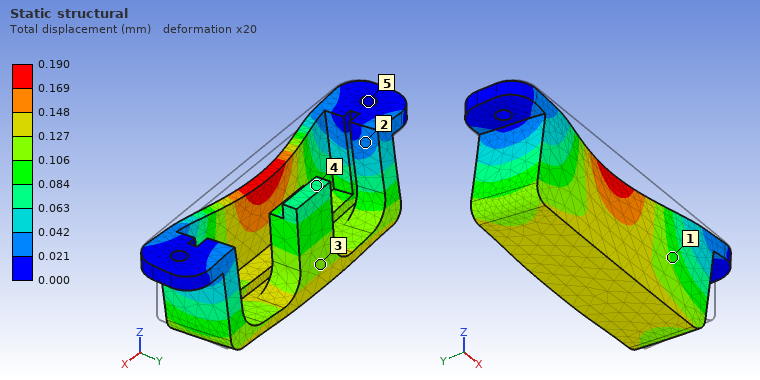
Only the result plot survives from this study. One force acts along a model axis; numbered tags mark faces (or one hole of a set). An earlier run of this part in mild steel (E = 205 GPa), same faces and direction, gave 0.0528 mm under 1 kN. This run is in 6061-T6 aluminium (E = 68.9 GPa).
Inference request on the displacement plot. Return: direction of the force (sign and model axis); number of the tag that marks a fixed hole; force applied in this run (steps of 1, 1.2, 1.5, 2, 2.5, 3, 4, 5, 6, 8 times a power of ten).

+Y
5
1.2 kN
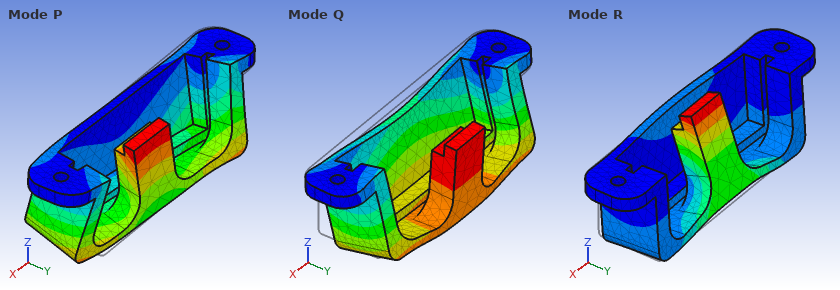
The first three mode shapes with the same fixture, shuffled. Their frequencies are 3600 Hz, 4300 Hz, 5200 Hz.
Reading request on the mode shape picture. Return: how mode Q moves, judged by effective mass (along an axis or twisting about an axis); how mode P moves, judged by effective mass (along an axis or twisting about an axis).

along Y
along X
